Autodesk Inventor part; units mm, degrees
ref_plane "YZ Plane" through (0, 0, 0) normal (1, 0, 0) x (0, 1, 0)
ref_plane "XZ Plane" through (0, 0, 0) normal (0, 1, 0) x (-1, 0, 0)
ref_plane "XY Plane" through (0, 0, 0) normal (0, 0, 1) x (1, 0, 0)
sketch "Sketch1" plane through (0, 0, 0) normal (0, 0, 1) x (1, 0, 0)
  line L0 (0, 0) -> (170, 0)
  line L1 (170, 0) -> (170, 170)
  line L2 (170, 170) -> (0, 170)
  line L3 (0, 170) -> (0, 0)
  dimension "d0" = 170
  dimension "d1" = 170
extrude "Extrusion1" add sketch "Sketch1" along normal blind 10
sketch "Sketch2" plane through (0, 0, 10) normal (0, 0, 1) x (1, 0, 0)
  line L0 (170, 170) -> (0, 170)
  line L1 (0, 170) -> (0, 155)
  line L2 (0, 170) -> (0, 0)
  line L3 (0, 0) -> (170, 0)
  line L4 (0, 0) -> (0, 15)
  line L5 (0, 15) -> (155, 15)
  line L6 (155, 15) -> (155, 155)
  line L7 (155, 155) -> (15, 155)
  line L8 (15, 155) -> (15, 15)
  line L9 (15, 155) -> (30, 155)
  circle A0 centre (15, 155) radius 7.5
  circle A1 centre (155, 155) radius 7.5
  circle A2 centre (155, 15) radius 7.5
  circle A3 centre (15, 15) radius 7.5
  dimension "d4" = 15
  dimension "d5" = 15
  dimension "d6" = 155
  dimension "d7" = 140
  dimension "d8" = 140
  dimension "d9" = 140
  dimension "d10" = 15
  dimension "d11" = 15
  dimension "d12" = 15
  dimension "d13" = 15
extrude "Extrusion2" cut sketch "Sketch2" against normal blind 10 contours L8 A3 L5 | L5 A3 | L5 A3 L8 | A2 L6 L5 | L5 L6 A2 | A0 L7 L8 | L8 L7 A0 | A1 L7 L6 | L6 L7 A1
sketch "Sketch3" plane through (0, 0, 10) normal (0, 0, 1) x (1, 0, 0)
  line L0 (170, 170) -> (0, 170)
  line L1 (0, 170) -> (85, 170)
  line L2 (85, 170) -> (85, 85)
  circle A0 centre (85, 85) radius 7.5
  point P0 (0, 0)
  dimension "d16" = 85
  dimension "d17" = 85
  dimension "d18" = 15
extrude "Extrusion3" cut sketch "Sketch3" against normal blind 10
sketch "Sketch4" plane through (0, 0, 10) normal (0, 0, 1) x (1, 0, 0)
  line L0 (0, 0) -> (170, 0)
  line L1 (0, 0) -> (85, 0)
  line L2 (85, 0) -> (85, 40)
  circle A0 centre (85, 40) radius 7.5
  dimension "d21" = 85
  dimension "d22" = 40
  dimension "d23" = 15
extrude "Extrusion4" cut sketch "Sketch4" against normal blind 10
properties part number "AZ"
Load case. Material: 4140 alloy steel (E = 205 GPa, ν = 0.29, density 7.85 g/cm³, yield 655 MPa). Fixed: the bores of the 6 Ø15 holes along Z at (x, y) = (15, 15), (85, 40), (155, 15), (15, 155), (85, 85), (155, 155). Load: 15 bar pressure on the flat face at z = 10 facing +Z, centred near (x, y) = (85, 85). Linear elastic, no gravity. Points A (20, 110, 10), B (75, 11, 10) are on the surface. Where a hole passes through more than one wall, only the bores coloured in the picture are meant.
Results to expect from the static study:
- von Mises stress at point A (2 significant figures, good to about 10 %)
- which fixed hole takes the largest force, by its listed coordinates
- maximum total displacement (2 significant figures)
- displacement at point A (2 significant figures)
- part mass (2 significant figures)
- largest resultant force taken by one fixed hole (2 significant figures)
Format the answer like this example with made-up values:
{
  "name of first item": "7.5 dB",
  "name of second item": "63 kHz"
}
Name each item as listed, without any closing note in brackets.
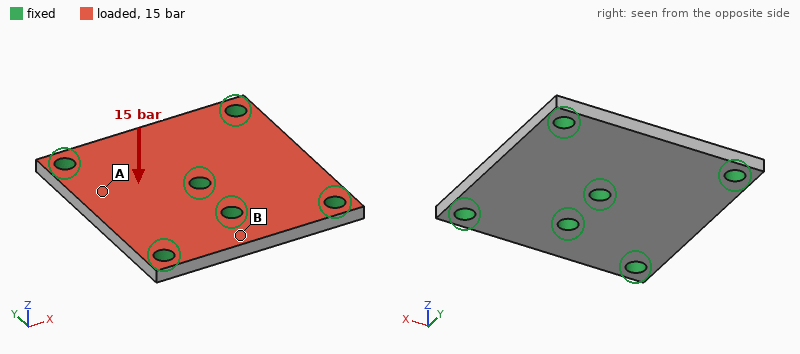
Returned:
{
  "von Mises stress at point A": "39 MPa",
  "which fixed hole takes the largest force, by its listed coordinates": "(85, 85)",
  "maximum total displacement": "60 µm",
  "displacement at point A": "37 µm",
  "part mass": "2.2 kg",
  "largest resultant force taken by one fixed hole": "11 kN"
}
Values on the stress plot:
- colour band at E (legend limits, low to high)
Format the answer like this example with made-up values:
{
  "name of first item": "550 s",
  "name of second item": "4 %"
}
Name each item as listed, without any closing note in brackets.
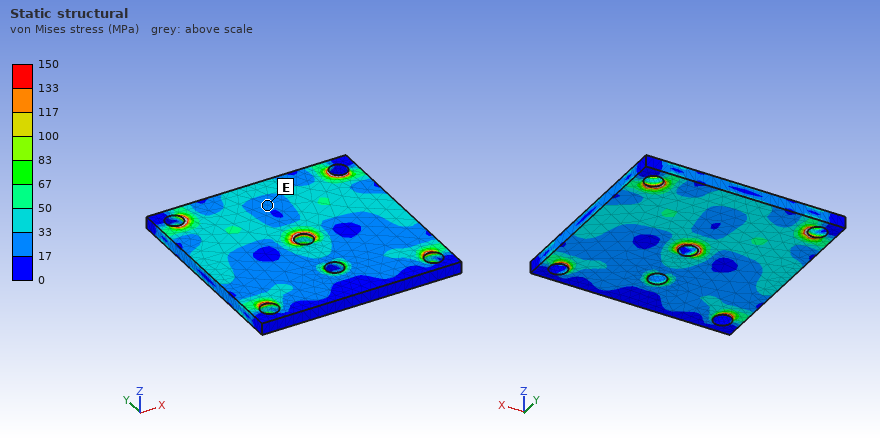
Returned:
{
  "colour band at E": "17 to 33 MPa"
}
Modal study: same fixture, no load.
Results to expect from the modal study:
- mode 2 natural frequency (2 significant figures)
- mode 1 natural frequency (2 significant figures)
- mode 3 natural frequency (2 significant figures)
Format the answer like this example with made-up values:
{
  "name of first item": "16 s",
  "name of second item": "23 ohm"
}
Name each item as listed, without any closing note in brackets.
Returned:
{
  "mode 2 natural frequency": "3600 Hz",
  "mode 1 natural frequency": "3500 Hz",
  "mode 3 natural frequency": "3700 Hz"
}
